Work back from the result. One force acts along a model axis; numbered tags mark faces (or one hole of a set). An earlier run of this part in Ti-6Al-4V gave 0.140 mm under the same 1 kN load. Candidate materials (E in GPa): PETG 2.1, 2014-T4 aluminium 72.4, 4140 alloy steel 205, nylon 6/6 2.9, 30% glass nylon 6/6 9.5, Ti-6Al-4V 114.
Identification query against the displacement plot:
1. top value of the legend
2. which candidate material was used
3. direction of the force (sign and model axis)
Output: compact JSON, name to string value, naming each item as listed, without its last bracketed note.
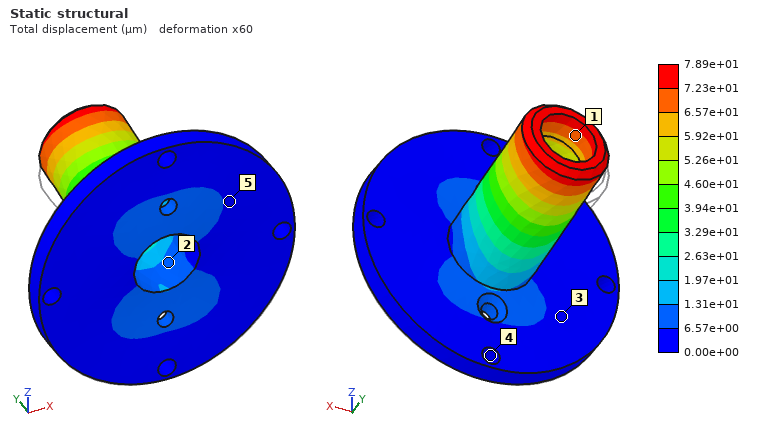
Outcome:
{"top value of the legend": "7.89e+01 µm", "which candidate material was used": "4140 alloy steel", "direction of the force": "+Z"}
